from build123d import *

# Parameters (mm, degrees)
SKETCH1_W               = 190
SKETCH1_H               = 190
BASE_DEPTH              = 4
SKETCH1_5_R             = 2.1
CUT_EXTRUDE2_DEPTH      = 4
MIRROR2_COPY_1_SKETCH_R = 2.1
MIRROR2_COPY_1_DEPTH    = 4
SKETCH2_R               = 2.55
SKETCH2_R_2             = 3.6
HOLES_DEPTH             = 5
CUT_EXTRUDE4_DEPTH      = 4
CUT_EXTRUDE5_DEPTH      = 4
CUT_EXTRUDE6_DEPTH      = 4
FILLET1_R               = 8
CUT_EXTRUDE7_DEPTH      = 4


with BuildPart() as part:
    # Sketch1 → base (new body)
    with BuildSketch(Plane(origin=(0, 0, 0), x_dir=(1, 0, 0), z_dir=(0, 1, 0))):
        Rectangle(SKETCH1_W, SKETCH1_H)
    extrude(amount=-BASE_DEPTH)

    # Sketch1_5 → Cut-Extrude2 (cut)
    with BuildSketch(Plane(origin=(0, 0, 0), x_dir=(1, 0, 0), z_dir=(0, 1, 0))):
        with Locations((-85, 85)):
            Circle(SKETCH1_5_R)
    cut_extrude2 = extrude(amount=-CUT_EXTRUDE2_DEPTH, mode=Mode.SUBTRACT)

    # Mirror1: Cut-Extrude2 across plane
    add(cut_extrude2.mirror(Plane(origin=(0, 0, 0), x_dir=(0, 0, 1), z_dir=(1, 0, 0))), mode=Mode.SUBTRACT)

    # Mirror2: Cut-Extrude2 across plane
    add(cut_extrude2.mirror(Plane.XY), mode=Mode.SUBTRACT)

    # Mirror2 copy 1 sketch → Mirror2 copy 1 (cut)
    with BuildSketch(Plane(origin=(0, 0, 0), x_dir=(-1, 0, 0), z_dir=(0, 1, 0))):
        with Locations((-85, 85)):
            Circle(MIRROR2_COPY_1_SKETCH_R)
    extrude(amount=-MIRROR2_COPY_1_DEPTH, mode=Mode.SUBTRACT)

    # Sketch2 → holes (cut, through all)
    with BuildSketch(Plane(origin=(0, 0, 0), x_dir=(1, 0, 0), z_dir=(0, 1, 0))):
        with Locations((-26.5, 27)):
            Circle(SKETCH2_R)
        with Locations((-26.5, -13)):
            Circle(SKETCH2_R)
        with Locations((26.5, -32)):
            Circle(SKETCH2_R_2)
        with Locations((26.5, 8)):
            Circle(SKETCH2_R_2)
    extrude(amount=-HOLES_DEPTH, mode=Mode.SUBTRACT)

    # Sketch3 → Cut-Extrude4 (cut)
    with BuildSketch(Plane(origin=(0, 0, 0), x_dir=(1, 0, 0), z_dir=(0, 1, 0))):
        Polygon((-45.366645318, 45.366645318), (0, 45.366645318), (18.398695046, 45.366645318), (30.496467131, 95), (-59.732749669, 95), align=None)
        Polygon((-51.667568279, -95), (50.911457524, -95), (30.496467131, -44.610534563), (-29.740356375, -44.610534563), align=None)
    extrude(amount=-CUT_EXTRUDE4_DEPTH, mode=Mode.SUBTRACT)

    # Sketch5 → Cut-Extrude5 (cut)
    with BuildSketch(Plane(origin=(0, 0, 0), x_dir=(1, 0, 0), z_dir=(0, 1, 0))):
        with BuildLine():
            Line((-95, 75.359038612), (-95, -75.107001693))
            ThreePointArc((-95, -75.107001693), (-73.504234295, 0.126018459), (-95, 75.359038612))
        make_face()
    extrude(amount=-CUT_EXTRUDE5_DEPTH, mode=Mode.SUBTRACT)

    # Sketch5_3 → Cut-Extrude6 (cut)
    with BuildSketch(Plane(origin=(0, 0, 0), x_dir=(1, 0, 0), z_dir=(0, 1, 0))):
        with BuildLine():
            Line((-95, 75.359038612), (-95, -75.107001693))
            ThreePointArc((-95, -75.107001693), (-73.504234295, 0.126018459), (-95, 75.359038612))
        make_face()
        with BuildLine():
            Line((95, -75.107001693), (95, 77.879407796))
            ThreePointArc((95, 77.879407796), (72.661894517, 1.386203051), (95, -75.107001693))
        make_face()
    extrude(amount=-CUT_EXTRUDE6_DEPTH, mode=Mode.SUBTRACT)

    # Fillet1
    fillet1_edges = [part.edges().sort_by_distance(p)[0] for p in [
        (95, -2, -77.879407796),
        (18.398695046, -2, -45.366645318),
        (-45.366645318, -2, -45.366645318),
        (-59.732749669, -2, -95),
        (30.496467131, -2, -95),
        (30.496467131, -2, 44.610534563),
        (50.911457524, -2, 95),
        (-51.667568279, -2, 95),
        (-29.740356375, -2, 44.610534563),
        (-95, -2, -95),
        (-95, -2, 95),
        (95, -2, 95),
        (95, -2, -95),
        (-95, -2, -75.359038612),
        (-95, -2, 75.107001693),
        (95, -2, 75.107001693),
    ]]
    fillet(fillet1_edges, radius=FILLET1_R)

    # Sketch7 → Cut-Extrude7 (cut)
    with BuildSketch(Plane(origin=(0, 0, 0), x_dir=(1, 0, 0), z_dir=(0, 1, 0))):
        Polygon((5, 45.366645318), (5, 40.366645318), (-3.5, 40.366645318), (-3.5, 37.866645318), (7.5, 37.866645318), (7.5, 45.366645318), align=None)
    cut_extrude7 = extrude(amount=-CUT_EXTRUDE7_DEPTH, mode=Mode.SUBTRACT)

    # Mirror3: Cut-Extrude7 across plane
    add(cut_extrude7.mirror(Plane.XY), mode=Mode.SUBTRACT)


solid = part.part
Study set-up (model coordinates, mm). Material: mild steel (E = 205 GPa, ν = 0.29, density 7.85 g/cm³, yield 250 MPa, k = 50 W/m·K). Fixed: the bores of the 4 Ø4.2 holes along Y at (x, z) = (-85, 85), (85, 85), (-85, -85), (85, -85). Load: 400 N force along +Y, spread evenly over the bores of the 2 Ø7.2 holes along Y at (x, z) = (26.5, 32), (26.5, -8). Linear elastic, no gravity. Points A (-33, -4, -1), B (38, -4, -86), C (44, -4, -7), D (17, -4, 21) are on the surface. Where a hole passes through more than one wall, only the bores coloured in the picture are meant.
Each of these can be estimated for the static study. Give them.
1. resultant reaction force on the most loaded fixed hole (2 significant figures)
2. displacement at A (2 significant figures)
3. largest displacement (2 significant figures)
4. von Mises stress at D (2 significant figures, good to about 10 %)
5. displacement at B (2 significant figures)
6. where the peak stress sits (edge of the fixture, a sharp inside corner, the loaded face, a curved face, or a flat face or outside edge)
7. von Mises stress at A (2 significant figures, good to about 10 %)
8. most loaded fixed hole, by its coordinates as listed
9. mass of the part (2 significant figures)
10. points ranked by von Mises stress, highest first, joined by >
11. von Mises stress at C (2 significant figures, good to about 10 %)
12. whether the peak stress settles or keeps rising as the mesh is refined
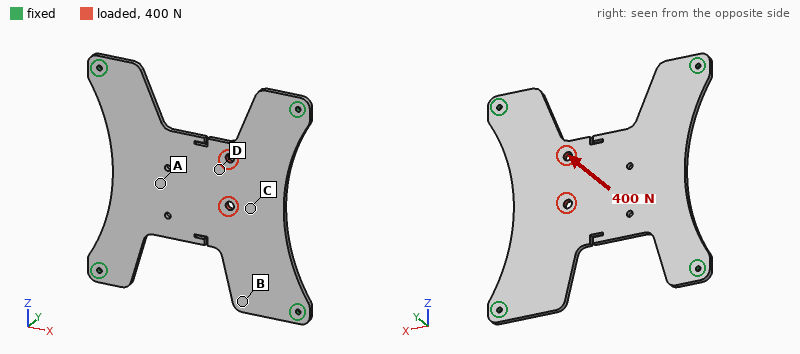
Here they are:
160 N
0.14 mm
0.21 mm
31 MPa
0.050 mm
edge of the fixture
11 MPa
(85, 85)
730 g
D > C > A > B
24 MPa
keeps rising
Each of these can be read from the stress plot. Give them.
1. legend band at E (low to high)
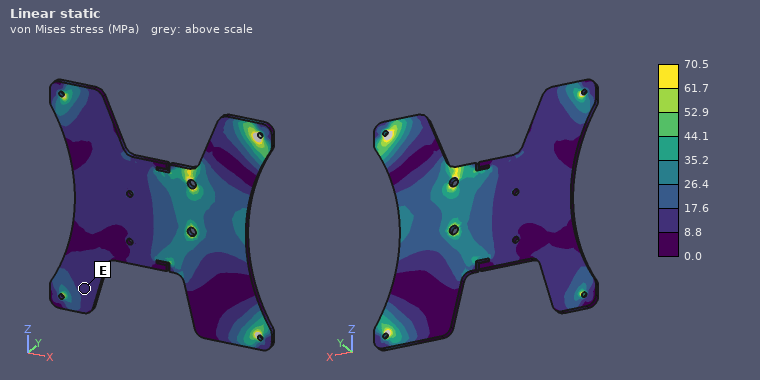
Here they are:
8.8 to 17.6 MPa
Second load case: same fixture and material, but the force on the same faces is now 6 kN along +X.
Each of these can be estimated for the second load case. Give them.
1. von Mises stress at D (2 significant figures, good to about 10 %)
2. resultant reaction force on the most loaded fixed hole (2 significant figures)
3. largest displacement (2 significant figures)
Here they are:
13 MPa
2.5 kN
15 µm
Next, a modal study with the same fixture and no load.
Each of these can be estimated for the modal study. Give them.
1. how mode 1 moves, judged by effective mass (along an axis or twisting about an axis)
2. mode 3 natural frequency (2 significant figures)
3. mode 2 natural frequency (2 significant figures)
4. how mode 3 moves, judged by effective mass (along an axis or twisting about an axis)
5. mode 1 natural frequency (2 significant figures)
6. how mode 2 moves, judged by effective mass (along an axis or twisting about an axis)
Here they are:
along Y
980 Hz
800 Hz
twisting about X
410 Hz
twisting about Z
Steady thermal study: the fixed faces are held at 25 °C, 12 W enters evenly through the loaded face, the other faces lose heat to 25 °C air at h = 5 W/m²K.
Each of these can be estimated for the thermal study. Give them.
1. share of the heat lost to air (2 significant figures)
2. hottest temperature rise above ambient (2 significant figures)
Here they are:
32 %
37 K
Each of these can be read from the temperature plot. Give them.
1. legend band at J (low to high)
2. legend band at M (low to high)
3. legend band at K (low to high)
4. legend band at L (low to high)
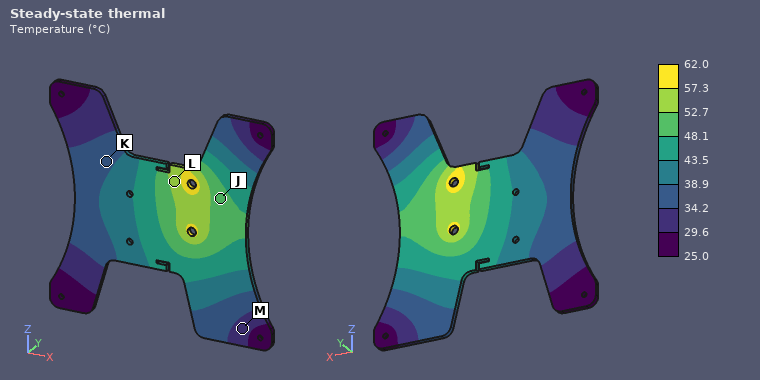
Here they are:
48.1 to 52.7 °C
29.6 to 34.2 °C
34.2 to 38.9 °C
52.7 to 57.3 °C
